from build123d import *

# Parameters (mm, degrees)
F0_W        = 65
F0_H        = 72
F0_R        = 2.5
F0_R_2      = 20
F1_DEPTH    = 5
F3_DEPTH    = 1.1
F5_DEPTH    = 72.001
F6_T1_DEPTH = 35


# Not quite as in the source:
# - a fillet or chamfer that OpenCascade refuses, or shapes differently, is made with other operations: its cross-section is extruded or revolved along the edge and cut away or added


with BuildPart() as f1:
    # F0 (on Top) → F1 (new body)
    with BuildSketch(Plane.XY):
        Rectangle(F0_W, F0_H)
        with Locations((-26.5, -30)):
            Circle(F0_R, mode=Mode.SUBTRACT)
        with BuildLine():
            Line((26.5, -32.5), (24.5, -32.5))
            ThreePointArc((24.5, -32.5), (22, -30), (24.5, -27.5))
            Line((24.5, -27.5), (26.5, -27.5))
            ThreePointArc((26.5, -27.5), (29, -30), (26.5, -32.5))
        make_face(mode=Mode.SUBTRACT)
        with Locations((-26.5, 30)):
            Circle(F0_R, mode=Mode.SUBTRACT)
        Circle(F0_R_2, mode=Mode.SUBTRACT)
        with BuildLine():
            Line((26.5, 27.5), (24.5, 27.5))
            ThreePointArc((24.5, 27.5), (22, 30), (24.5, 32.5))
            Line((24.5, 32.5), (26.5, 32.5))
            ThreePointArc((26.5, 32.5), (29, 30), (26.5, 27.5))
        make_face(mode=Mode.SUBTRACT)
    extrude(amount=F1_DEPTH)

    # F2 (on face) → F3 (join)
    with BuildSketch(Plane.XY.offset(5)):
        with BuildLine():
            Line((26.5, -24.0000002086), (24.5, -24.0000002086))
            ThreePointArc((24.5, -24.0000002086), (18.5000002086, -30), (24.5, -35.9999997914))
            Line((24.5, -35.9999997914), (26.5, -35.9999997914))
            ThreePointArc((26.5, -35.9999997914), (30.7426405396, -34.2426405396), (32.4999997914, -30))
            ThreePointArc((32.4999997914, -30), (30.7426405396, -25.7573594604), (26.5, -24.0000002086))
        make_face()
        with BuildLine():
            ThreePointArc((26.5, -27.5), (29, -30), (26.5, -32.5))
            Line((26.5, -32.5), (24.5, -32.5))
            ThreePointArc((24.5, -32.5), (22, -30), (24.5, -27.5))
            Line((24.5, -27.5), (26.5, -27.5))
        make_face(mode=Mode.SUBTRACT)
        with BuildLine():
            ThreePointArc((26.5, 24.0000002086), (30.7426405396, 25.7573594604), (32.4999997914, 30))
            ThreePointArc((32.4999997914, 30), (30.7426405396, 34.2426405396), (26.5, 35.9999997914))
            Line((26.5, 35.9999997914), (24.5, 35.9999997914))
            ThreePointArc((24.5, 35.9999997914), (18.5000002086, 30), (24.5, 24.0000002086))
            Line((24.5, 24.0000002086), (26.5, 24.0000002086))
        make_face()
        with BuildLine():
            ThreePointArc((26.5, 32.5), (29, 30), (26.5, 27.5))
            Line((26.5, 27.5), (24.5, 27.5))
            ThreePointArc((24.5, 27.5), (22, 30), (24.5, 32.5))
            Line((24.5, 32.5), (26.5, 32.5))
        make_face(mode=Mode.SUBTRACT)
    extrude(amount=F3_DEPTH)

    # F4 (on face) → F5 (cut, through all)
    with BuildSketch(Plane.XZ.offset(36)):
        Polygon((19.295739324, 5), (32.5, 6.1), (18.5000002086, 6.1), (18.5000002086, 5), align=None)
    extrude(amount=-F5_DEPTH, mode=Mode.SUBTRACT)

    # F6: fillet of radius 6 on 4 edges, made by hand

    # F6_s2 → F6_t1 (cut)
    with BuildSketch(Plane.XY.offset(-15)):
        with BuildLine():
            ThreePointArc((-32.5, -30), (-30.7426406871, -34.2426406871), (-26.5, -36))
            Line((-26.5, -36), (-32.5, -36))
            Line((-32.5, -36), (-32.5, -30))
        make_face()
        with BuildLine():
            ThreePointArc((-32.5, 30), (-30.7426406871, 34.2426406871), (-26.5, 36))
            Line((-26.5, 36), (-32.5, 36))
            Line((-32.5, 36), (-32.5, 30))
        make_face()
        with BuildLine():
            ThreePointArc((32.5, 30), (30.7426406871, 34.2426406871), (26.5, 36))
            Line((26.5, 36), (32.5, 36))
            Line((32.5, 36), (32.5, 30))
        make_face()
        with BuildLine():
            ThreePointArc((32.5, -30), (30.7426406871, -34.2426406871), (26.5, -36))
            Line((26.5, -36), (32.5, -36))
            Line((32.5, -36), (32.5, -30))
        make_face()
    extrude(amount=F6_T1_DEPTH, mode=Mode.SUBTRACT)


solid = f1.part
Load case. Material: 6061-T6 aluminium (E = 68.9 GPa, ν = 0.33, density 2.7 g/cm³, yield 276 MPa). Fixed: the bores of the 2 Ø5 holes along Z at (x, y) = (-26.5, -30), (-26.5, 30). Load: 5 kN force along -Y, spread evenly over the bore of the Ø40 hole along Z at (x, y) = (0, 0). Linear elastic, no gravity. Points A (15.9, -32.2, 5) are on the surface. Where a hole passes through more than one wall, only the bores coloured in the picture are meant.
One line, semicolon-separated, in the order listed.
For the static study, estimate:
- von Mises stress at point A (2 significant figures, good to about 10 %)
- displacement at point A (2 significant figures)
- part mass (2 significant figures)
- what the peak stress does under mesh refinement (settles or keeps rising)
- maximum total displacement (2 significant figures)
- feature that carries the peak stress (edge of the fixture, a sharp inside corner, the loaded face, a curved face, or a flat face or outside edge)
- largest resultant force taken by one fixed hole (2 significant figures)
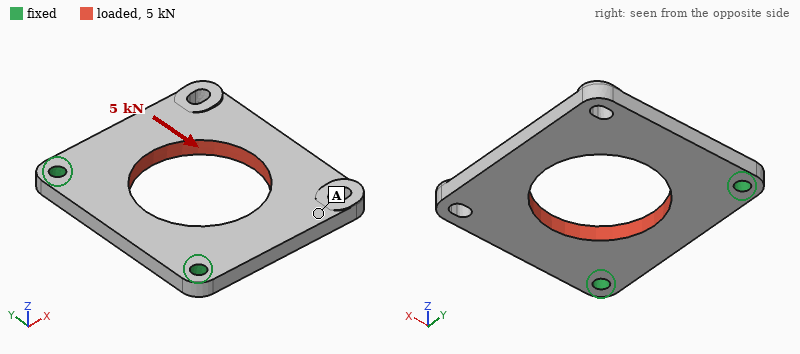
17 MPa; 0.095 mm; 45 g; keeps rising; 0.11 mm; edge of the fixture; 3.1 kN
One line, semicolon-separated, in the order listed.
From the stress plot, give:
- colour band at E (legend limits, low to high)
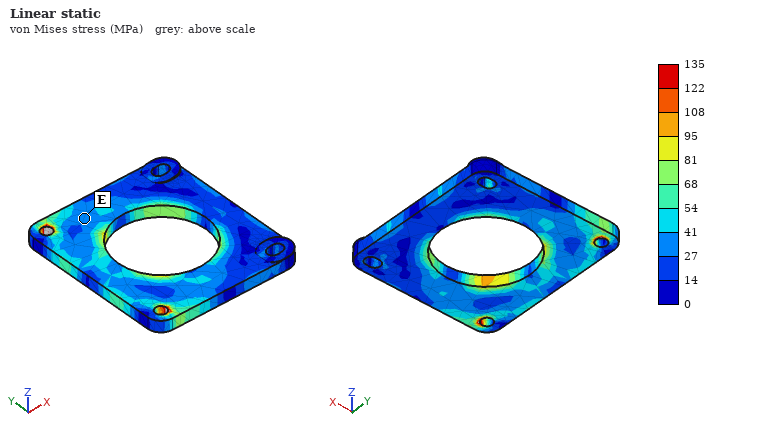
27 to 41 MPa
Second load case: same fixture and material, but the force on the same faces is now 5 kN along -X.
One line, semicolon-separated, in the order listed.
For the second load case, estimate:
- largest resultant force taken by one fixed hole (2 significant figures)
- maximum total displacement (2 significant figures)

2.6 kN; 23 µm
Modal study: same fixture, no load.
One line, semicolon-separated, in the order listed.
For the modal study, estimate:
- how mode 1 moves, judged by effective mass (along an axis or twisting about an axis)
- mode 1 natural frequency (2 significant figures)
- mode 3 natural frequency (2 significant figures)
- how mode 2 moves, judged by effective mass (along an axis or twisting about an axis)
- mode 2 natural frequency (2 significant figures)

along Z; 940 Hz; 5500 Hz; twisting about X; 2200 Hz
